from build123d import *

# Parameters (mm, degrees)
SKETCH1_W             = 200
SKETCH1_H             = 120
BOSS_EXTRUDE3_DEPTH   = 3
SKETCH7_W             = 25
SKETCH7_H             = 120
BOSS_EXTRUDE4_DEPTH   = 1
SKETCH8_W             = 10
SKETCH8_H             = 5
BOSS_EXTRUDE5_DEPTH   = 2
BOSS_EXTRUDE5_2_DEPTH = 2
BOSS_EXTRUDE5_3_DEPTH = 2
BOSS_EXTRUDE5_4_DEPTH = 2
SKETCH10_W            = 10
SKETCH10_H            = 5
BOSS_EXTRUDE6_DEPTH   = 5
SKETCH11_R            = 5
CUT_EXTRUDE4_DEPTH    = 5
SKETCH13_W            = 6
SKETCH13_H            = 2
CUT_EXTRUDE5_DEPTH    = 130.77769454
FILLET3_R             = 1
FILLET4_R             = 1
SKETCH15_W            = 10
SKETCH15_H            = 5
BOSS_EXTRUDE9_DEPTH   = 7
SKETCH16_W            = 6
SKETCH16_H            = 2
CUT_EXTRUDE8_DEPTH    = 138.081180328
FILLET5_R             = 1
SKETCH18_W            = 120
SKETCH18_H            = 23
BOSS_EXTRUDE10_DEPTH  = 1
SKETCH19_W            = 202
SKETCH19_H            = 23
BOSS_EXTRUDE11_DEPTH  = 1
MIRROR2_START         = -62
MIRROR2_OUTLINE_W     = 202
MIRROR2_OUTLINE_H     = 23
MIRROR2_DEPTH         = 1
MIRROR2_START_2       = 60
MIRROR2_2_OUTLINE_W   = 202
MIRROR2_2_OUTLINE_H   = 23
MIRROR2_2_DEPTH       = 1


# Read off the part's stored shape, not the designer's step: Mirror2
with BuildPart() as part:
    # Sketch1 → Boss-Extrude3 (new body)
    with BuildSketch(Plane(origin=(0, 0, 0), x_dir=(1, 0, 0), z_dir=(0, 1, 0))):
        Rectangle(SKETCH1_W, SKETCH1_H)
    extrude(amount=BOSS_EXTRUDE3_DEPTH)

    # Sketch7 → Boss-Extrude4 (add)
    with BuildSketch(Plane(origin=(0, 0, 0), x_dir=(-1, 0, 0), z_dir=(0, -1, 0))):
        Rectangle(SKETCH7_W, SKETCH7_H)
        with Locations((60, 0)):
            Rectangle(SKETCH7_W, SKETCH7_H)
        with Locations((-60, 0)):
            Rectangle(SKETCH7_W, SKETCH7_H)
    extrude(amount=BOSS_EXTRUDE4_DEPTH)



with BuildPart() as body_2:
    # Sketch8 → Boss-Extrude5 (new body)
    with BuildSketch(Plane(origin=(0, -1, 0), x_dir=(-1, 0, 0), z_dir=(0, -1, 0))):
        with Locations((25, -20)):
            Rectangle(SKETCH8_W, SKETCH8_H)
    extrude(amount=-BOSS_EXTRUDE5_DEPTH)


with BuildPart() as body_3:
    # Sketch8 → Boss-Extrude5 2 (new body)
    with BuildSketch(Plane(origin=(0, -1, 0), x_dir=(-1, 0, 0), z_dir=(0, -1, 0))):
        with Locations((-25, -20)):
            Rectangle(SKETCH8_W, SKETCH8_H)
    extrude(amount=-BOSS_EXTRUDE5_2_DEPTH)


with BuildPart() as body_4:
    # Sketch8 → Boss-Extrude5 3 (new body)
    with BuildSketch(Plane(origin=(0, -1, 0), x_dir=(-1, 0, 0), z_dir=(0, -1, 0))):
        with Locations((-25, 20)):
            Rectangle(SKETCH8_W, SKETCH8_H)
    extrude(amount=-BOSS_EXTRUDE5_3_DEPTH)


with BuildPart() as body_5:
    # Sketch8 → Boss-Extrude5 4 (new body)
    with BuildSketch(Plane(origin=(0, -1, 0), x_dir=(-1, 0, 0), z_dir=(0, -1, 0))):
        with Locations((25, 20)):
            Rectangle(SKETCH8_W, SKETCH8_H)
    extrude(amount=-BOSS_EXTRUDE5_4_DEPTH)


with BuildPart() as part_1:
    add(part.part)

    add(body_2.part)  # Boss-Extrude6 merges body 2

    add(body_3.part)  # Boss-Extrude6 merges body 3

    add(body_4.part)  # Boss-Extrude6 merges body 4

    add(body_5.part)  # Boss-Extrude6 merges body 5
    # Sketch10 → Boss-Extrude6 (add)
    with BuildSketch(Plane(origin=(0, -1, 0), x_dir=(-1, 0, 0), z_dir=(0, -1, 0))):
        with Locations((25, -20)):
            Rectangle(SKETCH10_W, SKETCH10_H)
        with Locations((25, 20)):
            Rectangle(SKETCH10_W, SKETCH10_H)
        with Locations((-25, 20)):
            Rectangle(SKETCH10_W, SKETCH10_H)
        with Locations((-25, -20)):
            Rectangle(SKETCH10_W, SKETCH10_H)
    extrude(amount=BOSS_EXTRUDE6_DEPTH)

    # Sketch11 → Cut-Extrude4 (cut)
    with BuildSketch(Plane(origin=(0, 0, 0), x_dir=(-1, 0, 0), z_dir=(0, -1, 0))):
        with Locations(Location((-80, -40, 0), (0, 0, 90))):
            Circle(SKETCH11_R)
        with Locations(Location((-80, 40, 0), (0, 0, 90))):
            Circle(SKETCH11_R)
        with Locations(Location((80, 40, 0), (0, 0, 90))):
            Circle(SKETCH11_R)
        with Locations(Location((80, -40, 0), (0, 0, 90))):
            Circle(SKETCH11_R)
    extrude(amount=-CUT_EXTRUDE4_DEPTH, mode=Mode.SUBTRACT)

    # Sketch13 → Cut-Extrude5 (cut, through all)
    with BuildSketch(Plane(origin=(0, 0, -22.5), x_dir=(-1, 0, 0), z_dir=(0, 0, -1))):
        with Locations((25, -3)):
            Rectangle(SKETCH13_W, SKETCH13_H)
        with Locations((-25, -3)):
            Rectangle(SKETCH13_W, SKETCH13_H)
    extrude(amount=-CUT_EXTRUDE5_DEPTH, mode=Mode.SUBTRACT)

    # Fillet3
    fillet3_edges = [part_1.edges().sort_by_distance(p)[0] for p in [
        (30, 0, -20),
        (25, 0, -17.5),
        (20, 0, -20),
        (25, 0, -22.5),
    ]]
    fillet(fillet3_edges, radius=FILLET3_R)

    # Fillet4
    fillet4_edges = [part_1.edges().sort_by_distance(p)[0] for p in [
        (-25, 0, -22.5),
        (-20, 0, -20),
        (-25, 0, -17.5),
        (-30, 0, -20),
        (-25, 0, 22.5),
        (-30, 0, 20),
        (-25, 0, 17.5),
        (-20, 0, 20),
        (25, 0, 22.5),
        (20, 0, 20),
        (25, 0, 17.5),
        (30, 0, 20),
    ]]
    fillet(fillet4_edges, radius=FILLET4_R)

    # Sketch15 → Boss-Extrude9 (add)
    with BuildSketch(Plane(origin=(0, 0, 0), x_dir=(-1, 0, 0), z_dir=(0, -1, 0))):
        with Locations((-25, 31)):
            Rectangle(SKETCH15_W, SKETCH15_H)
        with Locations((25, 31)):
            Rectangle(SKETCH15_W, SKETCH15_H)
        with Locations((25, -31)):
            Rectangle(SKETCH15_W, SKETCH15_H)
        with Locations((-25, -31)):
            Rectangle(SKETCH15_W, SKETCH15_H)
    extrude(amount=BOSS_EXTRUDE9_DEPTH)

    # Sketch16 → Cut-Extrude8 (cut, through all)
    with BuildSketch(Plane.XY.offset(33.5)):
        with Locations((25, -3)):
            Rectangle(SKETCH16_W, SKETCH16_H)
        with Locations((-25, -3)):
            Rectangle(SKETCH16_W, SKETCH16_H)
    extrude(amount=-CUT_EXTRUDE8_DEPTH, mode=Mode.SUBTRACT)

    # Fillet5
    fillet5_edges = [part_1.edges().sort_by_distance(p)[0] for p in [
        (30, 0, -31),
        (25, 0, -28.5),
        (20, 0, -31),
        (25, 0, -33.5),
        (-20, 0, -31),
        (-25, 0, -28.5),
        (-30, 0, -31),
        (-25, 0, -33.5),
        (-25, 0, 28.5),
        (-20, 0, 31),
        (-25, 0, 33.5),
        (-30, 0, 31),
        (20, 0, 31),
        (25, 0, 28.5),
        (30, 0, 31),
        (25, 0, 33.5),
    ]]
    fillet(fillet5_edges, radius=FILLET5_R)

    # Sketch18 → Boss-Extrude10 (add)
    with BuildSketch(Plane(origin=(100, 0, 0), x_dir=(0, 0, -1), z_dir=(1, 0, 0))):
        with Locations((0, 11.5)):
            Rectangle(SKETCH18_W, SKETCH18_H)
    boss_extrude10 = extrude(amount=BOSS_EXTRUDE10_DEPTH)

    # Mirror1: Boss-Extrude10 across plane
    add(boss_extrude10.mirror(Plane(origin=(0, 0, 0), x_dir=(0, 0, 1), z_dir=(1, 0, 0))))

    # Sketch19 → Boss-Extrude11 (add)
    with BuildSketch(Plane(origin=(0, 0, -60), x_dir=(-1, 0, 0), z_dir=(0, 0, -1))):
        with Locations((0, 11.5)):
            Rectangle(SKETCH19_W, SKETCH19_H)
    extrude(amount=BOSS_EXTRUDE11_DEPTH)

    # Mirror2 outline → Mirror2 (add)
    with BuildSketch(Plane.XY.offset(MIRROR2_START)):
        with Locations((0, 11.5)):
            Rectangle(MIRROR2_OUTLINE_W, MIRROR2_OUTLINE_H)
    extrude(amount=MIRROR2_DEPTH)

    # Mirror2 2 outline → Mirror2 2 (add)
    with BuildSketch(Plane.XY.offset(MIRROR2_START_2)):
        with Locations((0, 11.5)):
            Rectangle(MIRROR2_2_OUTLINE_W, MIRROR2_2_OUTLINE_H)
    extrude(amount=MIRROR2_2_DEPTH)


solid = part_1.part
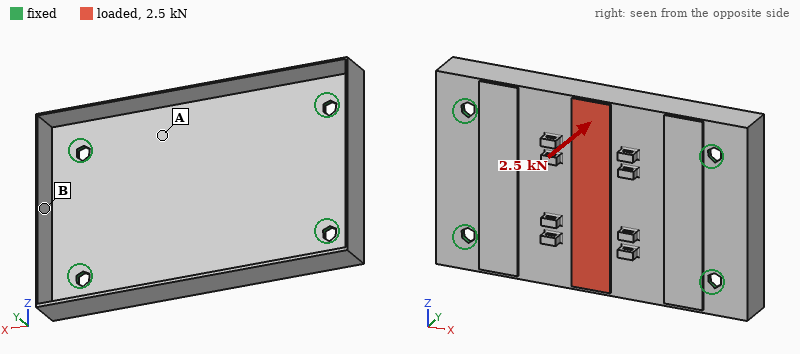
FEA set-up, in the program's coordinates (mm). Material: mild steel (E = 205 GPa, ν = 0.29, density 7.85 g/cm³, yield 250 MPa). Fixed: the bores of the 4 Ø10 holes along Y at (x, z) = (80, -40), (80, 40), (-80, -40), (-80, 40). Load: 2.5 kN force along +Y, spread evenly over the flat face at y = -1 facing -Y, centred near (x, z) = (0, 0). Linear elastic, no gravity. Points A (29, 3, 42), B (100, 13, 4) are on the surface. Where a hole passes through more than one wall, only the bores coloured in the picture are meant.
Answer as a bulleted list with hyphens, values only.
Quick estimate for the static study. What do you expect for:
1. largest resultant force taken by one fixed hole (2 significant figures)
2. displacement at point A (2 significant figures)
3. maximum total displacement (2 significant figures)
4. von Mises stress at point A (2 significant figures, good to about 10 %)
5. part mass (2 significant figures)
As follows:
- 970 N
- 0.16 mm
- 0.33 mm
- 56 MPa
- 800 g
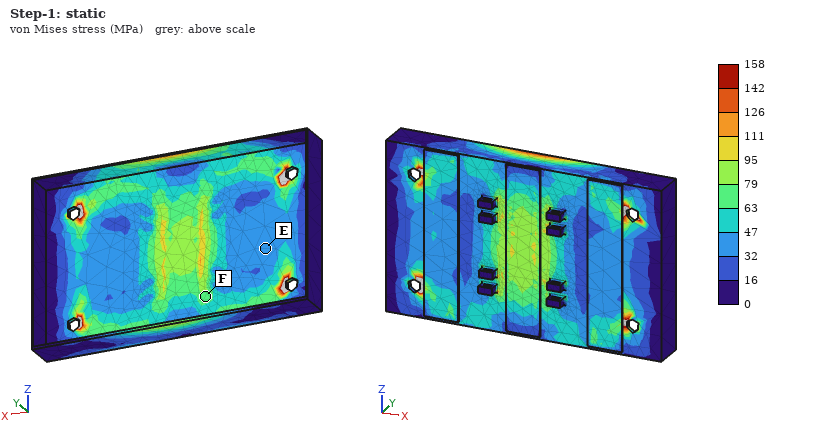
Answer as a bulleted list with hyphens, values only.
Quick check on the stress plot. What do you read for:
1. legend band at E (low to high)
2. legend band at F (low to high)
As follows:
- 32 to 47 MPa
- 63 to 79 MPa
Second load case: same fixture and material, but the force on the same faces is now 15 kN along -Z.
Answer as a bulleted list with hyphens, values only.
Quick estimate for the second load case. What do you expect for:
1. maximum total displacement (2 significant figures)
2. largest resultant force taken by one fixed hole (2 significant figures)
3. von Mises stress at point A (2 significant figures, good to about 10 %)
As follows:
- 31 µm
- 4.5 kN
- 33 MPa
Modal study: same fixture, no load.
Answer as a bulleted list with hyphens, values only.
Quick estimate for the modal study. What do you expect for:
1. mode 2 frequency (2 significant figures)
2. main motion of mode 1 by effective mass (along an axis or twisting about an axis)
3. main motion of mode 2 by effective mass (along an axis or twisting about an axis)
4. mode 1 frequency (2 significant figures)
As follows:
- 1700 Hz
- along Y
- twisting about X
- 970 Hz
